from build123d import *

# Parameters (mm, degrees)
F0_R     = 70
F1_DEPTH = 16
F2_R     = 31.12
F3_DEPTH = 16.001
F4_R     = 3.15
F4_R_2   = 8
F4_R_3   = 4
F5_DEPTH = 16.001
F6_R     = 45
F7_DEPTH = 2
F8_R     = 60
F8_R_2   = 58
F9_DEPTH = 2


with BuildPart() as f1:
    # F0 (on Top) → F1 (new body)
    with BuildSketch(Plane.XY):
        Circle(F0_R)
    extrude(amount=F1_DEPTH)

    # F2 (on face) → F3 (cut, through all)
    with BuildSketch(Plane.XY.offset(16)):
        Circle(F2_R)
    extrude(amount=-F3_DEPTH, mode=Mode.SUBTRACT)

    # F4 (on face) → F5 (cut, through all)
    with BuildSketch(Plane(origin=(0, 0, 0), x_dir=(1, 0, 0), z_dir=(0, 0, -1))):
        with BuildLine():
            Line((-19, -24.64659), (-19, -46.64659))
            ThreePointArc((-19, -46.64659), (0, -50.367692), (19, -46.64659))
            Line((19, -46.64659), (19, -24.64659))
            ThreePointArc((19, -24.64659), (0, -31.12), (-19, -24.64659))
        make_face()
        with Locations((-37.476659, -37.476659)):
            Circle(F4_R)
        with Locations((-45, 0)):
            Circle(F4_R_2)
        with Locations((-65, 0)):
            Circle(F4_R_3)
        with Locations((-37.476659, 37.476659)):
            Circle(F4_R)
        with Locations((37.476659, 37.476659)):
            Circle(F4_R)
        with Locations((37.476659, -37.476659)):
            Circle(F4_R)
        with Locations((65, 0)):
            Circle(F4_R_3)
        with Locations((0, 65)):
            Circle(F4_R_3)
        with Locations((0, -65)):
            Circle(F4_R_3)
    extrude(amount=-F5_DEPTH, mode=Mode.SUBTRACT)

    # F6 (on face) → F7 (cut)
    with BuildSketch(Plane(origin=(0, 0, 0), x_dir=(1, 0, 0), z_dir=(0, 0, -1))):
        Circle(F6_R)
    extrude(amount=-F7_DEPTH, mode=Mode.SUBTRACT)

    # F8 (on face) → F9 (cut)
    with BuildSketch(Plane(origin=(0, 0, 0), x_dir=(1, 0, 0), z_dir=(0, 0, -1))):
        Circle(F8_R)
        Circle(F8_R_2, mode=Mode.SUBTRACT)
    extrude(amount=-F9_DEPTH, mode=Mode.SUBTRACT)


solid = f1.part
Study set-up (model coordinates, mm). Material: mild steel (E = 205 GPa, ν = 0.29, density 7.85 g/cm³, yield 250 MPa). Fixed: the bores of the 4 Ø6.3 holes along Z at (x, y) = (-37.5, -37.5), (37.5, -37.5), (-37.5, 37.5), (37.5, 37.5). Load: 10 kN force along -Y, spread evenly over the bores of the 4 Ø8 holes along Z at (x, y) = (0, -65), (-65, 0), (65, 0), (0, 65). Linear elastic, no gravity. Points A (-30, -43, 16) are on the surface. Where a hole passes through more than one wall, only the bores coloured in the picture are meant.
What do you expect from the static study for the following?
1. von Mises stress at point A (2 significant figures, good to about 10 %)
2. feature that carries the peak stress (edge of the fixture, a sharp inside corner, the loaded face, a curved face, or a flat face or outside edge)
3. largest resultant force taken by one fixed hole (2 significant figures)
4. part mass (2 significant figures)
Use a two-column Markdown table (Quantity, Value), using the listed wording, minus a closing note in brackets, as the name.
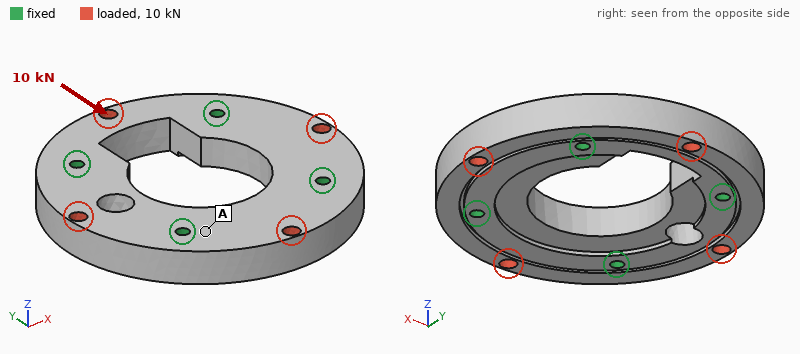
| Quantity | Value |
|---|---|
| von Mises stress at point A | 5.6 MPa |
| feature that carries the peak stress | a curved face |
| largest resultant force taken by one fixed hole | 2.9 kN |
| part mass | 1.3 kg |
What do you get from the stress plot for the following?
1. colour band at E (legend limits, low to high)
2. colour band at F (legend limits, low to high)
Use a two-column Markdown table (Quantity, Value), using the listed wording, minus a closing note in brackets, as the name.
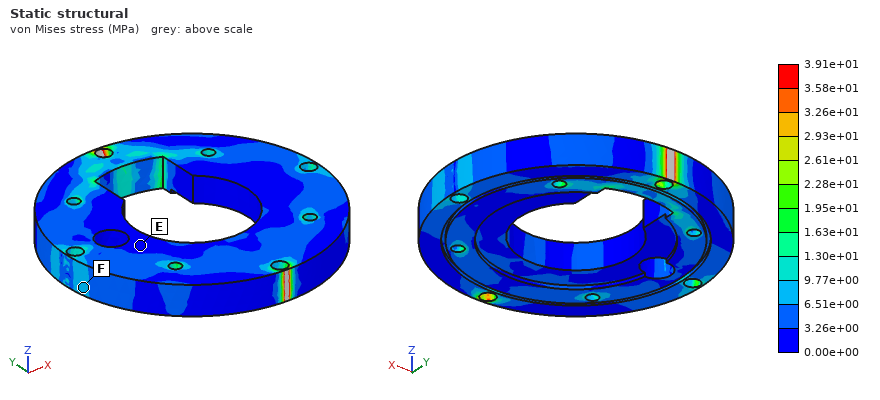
| Quantity | Value |
|---|---|
| colour band at E | 0.00e+00 to 3.26e+00 MPa |
| colour band at F | 6.51e+00 to 9.77e+00 MPa |
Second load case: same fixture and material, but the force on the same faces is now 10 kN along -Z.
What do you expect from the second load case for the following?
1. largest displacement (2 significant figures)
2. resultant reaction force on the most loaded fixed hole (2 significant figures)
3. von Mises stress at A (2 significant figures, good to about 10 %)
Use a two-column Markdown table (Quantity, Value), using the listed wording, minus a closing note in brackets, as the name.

| Quantity | Value |
|---|---|
| largest displacement | 18 µm |
| resultant reaction force on the most loaded fixed hole | 2.5 kN |
| von Mises stress at A | 23 MPa |
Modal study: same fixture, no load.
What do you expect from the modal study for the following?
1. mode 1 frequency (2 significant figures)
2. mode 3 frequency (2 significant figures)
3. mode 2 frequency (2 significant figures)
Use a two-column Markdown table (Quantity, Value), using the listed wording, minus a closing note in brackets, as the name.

| Quantity | Value |
|---|---|
| mode 1 frequency | 7000 Hz |
| mode 3 frequency | 7800 Hz |
| mode 2 frequency | 7800 Hz |
